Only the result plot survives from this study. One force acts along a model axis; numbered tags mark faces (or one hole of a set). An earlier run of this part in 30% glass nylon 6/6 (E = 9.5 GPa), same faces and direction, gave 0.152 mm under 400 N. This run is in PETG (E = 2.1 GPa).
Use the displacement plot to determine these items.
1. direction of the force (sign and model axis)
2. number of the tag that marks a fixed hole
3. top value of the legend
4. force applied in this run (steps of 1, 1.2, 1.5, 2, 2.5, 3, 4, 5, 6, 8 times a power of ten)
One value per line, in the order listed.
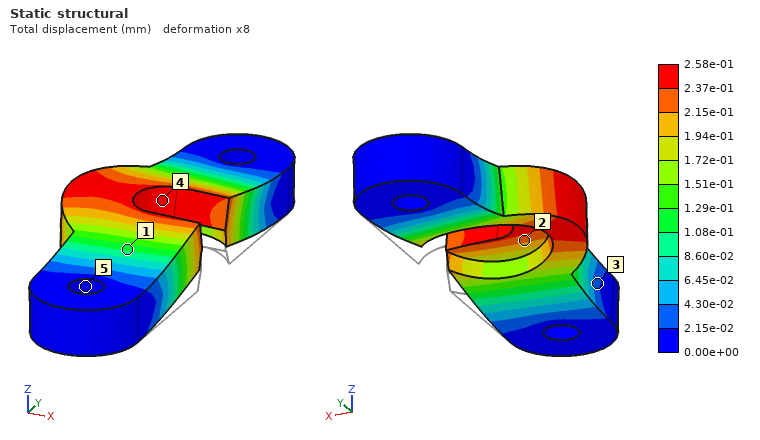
+Z
5
2.58e-01 mm
150 N
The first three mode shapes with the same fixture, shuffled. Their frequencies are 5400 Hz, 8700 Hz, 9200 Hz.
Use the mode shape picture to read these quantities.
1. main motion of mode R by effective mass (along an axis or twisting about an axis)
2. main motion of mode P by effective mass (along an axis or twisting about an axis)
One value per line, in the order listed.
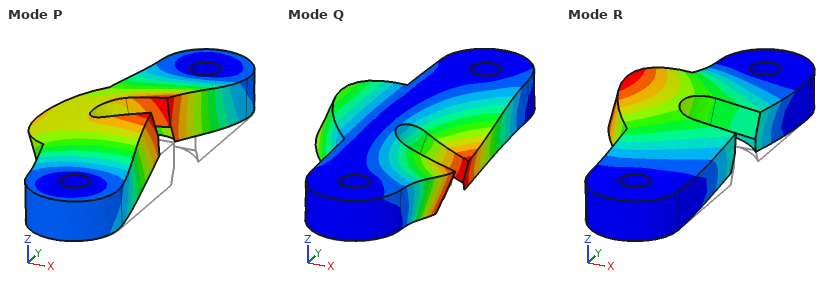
along Z
along X
